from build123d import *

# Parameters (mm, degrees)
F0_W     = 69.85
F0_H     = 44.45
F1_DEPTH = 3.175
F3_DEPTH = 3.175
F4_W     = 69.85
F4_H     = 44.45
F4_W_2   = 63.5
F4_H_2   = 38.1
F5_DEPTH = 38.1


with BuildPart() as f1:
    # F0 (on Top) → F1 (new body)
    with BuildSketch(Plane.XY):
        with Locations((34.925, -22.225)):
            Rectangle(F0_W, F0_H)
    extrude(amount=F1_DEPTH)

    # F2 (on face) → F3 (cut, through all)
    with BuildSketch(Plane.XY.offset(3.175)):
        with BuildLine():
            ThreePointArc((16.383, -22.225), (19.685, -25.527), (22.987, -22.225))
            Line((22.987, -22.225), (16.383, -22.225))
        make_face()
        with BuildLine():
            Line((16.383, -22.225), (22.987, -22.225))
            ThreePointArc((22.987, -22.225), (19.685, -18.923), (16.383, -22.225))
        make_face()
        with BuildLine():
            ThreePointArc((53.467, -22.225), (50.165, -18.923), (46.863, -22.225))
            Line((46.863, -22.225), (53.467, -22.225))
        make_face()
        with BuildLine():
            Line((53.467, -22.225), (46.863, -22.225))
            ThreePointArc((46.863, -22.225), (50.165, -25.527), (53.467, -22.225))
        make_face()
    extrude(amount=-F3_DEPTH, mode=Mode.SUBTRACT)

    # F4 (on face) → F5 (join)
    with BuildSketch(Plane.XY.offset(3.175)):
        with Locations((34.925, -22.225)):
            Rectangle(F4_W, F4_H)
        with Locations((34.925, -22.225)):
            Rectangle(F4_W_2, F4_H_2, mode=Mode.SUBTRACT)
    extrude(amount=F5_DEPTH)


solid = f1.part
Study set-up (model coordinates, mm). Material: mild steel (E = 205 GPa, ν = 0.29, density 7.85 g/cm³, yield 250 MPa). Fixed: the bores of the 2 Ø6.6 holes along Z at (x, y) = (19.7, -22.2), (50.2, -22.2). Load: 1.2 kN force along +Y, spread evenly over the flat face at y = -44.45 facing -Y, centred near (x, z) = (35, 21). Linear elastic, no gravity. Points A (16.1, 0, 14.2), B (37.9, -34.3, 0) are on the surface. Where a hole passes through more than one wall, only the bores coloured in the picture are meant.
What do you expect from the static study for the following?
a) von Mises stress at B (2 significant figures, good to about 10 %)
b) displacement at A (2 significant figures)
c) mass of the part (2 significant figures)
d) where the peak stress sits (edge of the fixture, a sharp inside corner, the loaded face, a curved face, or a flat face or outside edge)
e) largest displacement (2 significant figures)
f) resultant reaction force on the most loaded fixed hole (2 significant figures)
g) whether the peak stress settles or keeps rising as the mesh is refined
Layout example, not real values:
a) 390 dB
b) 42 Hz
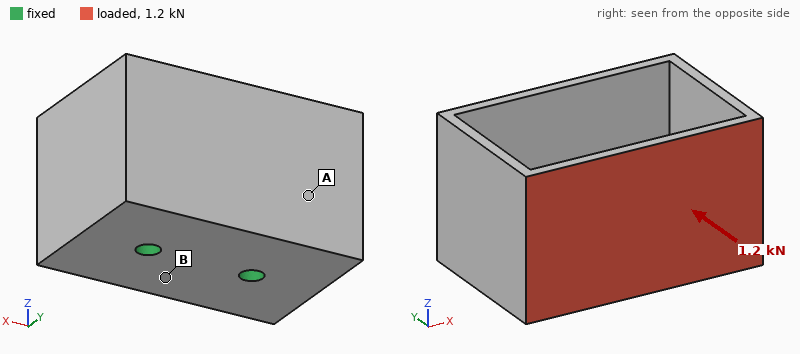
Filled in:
a) 44 MPa
b) 0.053 mm
c) 280 g
d) edge of the fixture
e) 0.15 mm
f) 610 N
g) keeps rising
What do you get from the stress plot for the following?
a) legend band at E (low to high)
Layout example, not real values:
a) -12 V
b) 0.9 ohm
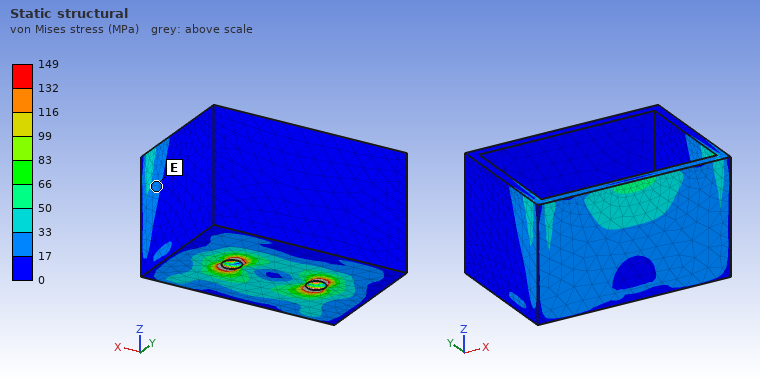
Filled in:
a) 17 to 33 MPa
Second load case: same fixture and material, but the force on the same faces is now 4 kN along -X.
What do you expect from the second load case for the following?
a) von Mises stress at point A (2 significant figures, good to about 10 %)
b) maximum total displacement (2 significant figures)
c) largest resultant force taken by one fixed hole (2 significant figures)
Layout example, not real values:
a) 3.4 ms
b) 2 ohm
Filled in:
a) 29 MPa
b) 0.17 mm
c) 3.6 kN
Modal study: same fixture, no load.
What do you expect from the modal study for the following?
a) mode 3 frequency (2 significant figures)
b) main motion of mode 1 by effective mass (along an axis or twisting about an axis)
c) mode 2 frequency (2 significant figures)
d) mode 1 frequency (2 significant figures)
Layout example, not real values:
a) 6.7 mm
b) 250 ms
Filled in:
a) 2100 Hz
b) along Y
c) 2000 Hz
d) 1200 Hz
